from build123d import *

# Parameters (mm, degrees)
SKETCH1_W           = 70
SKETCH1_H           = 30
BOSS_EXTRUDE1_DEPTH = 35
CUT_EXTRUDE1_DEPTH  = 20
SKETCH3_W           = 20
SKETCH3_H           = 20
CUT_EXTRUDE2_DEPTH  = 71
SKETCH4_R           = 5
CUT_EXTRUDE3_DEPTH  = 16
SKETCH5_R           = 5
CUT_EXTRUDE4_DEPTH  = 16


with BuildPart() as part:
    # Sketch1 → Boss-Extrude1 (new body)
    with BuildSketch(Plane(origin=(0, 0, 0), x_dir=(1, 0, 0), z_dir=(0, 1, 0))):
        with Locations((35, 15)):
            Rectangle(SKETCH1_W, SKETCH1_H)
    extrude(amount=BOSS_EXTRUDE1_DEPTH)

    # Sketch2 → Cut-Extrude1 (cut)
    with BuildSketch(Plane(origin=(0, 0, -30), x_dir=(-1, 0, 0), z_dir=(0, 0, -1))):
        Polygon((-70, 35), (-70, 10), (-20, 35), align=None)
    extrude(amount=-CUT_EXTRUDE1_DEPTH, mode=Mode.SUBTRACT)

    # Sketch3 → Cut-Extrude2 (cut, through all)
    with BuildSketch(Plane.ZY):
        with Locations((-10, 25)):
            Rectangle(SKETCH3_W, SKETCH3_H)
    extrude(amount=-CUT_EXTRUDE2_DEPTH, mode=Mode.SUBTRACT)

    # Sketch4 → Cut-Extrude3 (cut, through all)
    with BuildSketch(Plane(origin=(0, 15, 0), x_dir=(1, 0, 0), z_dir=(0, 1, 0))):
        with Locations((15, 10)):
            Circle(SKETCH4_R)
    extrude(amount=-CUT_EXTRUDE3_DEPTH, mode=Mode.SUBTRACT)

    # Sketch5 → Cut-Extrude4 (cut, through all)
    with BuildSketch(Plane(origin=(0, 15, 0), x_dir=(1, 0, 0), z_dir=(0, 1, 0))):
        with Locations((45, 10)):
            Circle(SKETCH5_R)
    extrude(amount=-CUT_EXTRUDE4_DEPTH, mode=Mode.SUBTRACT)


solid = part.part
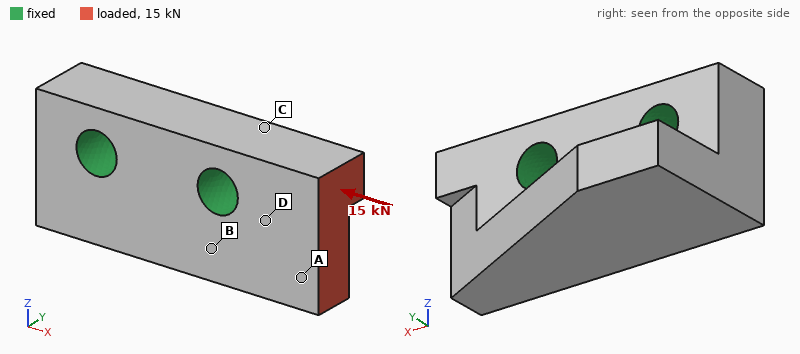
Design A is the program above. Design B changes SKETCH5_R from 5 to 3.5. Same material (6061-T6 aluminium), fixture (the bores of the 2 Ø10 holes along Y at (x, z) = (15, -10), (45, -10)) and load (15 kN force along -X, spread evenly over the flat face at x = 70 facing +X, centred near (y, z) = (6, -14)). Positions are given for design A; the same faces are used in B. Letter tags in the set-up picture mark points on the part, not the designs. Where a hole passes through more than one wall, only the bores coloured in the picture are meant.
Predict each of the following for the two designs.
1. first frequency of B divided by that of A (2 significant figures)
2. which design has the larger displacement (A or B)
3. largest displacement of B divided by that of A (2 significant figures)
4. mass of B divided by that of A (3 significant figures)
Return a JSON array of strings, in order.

["0.99", "B", "1.1", "1.02"]
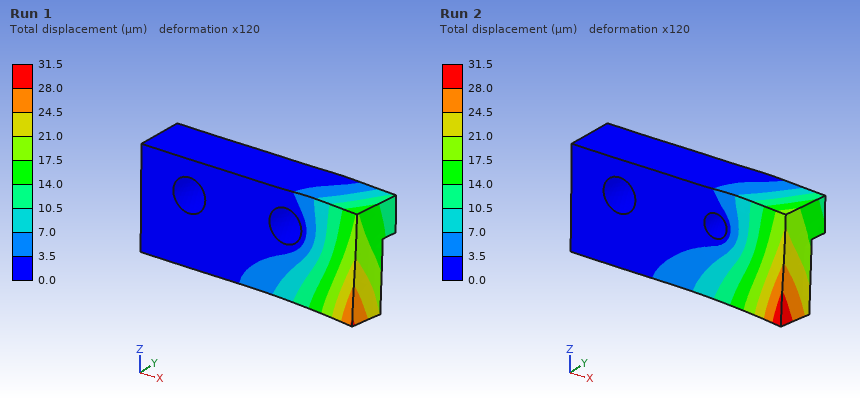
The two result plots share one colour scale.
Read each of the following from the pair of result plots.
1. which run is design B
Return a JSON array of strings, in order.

["Run 2"]
